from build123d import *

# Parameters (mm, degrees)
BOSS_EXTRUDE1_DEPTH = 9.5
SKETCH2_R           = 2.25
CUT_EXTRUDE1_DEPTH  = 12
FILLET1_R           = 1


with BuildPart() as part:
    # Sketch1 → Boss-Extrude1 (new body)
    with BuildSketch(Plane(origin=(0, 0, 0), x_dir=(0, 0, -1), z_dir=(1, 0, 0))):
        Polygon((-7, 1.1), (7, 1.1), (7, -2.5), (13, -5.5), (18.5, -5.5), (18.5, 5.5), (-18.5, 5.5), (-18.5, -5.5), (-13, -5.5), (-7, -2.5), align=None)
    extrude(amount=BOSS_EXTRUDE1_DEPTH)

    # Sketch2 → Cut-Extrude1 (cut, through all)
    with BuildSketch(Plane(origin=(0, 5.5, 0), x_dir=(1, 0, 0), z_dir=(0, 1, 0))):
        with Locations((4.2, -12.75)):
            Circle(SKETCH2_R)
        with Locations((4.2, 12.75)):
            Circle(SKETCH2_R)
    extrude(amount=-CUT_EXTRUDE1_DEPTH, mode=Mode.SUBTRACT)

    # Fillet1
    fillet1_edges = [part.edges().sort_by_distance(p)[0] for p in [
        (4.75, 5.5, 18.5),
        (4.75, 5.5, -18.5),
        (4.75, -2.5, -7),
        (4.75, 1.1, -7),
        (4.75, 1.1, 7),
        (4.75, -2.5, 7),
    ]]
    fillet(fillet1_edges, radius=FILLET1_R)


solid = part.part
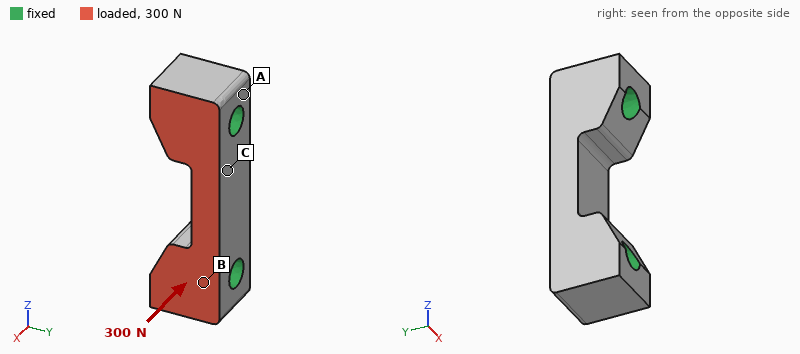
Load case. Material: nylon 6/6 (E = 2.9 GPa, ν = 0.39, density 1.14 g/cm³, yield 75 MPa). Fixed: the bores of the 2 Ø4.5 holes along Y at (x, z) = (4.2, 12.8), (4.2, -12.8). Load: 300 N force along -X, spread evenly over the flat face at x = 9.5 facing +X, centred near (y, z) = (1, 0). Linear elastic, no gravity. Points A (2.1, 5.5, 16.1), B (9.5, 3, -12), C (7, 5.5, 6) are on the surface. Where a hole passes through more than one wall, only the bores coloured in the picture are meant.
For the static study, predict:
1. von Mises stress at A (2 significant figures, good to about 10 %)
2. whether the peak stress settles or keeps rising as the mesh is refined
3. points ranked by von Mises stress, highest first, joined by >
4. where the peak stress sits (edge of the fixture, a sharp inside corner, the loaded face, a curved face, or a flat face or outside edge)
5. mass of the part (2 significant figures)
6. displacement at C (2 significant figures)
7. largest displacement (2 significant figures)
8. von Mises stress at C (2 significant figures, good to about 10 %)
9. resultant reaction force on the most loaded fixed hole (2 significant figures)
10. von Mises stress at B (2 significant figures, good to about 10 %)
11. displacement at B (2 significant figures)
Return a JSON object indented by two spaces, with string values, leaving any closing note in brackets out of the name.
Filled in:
{
  "von Mises stress at A": "0.65 MPa",
  "whether the peak stress settles or keeps rising as the mesh is refined": "keeps rising",
  "points ranked by von Mises stress, highest first, joined by >": "B > C > A",
  "where the peak stress sits": "edge of the fixture",
  "mass of the part": "2.8 g",
  "displacement at C": "8.0 µm",
  "largest displacement": "12 µm",
  "von Mises stress at C": "1.5 MPa",
  "resultant reaction force on the most loaded fixed hole": "150 N",
  "von Mises stress at B": "2.3 MPa",
  "displacement at B": "2.2 µm"
}
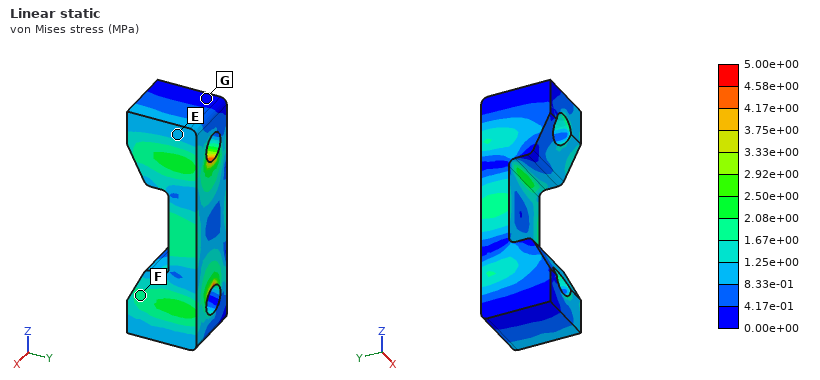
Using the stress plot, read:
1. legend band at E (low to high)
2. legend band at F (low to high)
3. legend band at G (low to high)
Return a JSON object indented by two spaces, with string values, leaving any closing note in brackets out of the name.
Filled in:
{
  "legend band at E": "8.33e-01 to 1.25e+00 MPa",
  "legend band at F": "1.67e+00 to 2.08e+00 MPa",
  "legend band at G": "0.00e+00 to 4.17e-01 MPa"
}
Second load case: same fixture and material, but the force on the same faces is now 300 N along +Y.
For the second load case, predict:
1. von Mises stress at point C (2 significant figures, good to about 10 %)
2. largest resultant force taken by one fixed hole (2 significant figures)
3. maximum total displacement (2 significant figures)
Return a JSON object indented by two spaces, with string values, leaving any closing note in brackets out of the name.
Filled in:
{
  "von Mises stress at point C": "3.3 MPa",
  "largest resultant force taken by one fixed hole": "150 N",
  "maximum total displacement": "35 µm"
}
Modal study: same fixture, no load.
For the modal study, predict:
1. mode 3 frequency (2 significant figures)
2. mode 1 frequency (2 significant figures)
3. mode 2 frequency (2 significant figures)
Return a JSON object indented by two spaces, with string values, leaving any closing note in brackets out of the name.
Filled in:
{
  "mode 3 frequency": "22 kHz",
  "mode 1 frequency": "16 kHz",
  "mode 2 frequency": "17 kHz"
}
